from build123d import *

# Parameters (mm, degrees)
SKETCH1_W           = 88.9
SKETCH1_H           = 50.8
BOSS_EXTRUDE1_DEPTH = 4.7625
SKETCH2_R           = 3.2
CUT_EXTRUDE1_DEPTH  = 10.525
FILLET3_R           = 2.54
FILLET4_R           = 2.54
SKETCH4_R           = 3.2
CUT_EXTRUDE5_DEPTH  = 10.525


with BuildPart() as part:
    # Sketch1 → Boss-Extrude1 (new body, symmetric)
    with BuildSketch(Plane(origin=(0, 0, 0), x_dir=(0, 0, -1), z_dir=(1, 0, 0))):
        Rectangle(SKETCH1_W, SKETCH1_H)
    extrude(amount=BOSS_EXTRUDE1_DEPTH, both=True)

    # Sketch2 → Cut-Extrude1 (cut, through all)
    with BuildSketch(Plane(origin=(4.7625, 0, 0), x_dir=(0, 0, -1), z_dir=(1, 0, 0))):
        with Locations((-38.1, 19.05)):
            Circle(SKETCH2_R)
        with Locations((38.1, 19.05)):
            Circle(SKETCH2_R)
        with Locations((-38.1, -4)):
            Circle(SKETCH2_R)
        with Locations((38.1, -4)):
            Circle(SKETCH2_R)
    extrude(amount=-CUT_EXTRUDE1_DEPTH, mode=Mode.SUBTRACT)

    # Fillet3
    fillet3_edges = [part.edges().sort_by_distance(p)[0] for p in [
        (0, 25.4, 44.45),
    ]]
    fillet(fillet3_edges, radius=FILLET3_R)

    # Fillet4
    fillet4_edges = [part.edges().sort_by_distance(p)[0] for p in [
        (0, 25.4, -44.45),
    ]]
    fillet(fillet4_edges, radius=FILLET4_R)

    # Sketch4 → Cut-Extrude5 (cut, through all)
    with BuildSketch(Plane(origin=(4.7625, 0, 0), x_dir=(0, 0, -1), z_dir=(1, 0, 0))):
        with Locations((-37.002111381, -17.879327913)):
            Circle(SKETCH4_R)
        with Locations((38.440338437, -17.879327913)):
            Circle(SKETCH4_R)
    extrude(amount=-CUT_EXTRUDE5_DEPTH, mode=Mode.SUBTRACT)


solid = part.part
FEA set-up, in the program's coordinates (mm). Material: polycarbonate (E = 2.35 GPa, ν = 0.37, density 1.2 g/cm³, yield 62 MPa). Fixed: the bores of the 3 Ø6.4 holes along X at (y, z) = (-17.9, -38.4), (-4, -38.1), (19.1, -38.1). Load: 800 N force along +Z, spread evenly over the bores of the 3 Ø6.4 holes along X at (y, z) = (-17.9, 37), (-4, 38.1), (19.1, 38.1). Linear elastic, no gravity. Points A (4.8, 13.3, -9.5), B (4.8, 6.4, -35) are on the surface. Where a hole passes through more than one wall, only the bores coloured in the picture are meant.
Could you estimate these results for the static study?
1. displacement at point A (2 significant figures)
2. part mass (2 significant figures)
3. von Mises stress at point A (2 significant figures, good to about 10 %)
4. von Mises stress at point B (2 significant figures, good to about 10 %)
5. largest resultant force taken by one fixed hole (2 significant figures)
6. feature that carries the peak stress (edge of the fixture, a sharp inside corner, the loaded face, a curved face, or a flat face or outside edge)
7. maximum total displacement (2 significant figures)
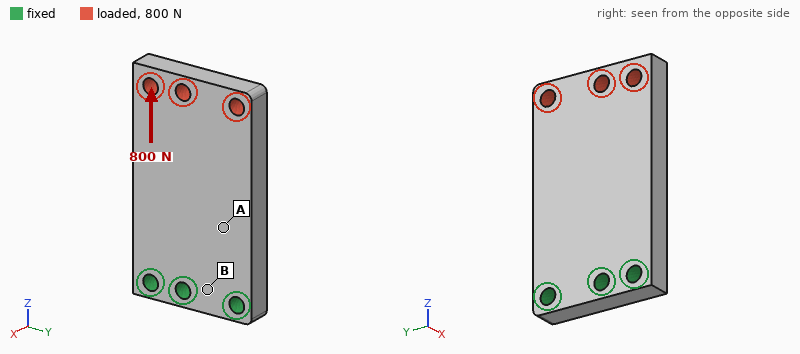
19 µm
49 g
1.5 MPa
0.54 MPa
280 N
the loaded face
66 µm
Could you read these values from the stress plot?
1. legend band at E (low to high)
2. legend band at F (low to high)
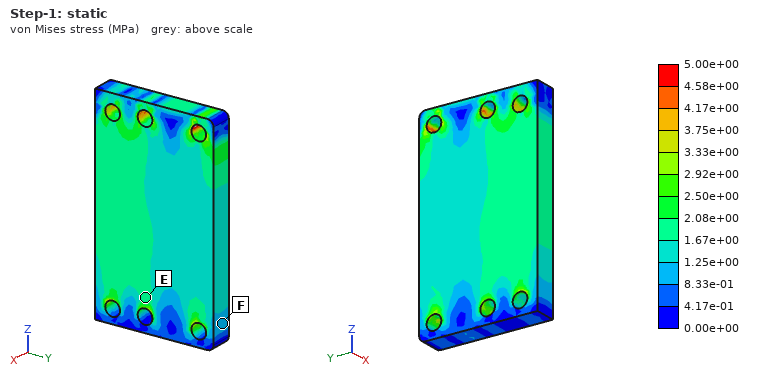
1.67e+00 to 2.08e+00 MPa
8.33e-01 to 1.25e+00 MPa
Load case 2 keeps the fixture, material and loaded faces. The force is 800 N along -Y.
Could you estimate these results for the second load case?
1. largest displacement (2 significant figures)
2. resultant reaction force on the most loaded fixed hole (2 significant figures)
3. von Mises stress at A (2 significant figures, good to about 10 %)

0.76 mm
1.6 kN
5.9 MPa
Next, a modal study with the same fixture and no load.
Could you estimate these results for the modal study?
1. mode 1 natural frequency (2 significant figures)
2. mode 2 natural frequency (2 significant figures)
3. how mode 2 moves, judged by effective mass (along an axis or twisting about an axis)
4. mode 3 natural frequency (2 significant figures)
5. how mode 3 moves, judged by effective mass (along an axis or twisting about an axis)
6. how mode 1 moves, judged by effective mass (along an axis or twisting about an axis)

340 Hz
1100 Hz
twisting about Z
1400 Hz
along Y
along X
